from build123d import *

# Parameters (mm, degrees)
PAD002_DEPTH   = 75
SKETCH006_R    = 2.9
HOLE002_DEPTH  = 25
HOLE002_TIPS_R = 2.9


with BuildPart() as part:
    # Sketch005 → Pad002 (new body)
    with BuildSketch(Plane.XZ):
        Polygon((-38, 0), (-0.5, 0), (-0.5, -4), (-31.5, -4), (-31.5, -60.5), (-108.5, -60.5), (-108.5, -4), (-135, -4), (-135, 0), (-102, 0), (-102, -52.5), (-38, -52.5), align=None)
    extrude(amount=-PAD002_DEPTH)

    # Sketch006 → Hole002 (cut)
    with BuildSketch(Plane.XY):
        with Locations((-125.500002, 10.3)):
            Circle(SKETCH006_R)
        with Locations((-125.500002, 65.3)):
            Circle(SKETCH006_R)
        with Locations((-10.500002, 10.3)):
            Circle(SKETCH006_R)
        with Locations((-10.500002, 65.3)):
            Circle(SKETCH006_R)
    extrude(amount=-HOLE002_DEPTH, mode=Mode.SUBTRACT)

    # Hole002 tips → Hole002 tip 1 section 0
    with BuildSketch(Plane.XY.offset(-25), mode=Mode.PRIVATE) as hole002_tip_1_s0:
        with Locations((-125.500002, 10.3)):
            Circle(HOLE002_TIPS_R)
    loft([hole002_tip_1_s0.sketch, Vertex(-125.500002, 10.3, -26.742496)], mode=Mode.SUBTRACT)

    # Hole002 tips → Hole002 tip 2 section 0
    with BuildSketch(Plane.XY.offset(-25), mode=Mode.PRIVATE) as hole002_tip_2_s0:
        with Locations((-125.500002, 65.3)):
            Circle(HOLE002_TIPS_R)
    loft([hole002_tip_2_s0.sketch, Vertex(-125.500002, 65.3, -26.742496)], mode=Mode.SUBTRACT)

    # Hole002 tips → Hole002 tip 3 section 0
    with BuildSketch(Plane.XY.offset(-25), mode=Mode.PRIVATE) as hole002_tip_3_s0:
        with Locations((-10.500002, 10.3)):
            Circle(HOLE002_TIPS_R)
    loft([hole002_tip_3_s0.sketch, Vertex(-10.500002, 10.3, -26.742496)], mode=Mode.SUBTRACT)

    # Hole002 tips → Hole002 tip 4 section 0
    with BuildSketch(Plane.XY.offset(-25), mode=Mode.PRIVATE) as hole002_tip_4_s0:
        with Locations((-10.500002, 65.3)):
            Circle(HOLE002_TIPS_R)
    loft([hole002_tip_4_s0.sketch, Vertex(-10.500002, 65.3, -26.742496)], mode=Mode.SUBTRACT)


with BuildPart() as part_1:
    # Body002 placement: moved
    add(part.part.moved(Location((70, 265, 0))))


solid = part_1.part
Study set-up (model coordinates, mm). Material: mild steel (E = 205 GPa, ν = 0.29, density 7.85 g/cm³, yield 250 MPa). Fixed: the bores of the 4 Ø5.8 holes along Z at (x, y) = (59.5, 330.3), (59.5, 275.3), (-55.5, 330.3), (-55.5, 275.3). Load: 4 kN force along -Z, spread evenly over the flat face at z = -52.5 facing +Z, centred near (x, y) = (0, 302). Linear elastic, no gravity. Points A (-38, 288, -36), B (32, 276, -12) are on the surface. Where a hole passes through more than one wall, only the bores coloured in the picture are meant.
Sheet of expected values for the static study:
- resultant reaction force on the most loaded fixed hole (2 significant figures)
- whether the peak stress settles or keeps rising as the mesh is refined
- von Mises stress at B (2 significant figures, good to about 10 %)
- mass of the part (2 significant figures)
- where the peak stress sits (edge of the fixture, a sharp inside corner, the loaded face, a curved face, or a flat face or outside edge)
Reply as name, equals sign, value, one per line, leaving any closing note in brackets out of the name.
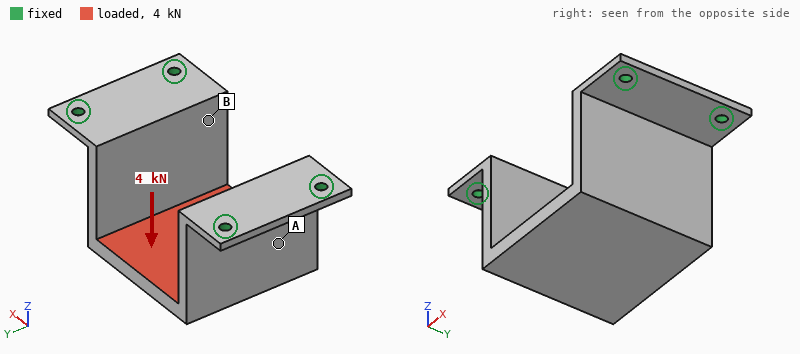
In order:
resultant reaction force on the most loaded fixed hole = 1.1 kN
whether the peak stress settles or keeps rising as the mesh is refined = keeps rising
von Mises stress at B = 27 MPa
mass of the part = 900 g
where the peak stress sits = edge of the fixture
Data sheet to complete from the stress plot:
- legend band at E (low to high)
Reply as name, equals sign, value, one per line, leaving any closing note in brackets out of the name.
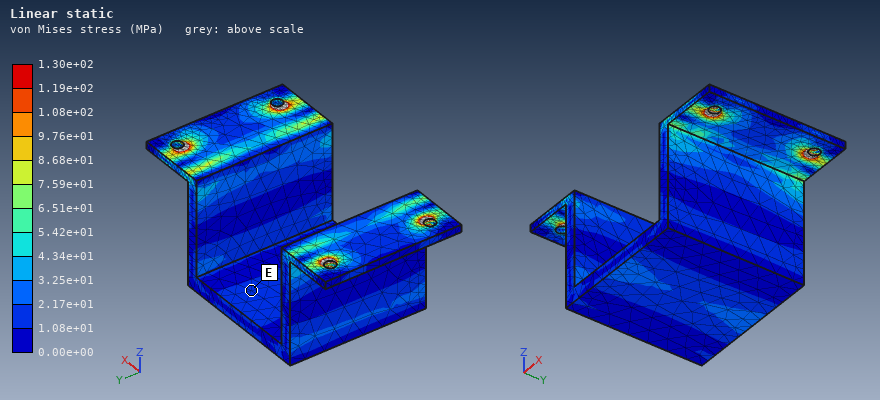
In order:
legend band at E = 1.08e+01 to 2.17e+01 MPa
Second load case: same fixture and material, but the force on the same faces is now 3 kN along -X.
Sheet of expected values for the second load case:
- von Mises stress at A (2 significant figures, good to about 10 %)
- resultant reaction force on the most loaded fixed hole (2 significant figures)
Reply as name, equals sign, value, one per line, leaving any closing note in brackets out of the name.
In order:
von Mises stress at A = 40 MPa
resultant reaction force on the most loaded fixed hole = 1.1 kN
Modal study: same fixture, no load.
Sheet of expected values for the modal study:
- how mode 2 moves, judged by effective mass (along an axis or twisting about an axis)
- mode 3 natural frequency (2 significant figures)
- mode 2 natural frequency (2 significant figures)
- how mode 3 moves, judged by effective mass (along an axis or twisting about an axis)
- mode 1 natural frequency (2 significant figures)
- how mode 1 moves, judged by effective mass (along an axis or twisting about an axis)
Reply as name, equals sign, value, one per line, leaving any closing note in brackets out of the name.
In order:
how mode 2 moves, judged by effective mass = along Y
mode 3 natural frequency = 1800 Hz
mode 2 natural frequency = 1100 Hz
how mode 3 moves, judged by effective mass = twisting about Z
mode 1 natural frequency = 1100 Hz
how mode 1 moves, judged by effective mass = along X
